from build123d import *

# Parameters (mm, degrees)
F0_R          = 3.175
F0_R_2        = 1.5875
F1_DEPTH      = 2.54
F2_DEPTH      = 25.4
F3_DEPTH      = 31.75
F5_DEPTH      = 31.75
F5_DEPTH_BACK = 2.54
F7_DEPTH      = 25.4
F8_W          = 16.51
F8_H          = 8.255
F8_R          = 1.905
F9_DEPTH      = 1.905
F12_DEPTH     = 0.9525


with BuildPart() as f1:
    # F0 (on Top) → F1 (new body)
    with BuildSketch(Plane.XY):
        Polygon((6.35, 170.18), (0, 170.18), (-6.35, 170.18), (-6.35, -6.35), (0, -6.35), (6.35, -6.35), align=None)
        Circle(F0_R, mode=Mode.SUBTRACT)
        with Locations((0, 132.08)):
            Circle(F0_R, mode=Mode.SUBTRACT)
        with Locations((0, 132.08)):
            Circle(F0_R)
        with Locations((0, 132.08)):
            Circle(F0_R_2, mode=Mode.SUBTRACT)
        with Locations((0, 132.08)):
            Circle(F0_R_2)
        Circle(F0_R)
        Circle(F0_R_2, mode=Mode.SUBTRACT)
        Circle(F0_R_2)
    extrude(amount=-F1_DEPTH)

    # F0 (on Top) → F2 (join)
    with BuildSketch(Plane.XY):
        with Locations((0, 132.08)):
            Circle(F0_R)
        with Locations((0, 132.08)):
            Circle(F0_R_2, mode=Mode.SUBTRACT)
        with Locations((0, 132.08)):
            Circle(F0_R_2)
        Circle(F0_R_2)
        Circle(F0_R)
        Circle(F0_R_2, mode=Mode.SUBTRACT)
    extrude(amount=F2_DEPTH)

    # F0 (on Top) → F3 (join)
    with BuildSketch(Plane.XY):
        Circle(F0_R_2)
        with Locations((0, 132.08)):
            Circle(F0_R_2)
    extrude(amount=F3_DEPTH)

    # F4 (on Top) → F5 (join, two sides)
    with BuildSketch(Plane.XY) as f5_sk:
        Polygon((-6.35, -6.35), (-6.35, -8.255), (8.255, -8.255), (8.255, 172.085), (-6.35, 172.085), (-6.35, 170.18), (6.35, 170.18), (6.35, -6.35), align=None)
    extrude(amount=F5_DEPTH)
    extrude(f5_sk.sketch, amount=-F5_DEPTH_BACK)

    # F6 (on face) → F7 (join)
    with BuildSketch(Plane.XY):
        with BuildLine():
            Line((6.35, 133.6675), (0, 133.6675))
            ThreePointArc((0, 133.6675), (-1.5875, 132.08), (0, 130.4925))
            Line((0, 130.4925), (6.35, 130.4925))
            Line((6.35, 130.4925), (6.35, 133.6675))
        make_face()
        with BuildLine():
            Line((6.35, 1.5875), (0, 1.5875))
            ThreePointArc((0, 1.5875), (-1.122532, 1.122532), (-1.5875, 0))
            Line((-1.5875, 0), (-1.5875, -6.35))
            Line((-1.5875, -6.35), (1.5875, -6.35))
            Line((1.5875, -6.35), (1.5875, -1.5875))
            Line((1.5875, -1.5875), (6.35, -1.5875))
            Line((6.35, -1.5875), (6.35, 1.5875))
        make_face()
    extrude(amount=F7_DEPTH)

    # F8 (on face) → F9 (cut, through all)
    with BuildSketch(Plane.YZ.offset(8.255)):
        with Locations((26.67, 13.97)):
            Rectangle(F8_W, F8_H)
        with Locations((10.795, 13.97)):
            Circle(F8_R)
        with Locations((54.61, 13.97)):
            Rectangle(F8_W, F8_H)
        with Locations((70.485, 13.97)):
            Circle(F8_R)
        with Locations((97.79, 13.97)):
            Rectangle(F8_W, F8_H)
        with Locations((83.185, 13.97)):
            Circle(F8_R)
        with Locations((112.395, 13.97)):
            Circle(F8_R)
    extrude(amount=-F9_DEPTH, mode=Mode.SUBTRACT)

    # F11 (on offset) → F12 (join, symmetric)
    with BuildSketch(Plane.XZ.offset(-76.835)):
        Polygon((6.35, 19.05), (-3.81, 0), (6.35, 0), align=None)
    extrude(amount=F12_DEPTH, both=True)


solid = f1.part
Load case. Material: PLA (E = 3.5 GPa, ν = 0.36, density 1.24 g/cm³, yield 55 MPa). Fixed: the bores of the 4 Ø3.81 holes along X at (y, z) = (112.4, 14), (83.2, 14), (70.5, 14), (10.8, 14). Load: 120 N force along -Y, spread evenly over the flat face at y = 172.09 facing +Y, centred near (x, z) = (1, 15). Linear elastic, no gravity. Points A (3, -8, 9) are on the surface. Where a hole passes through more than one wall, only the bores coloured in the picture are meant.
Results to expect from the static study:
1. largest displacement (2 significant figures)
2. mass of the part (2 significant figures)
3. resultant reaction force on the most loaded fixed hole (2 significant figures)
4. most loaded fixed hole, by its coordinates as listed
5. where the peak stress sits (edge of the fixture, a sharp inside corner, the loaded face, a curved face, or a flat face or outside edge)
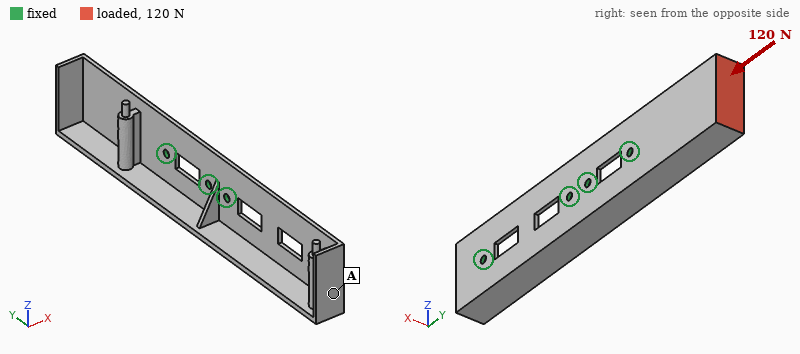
1.9 mm
26 g
55 N
(112.4, 14)
the loaded face
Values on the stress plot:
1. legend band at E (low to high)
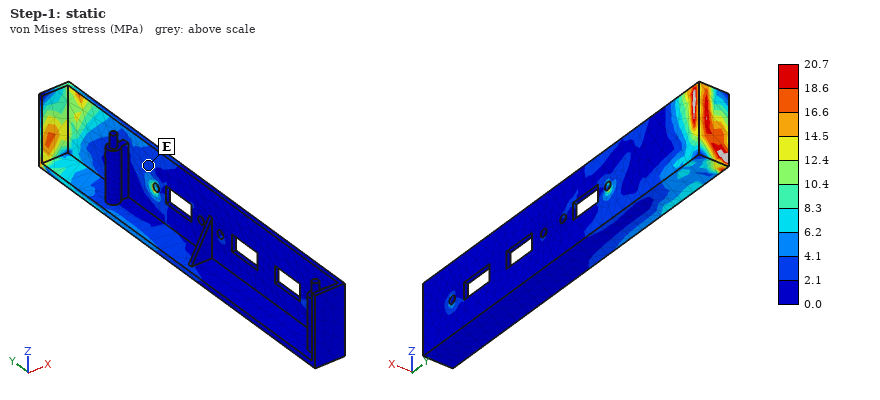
2.1 to 4.1 MPa
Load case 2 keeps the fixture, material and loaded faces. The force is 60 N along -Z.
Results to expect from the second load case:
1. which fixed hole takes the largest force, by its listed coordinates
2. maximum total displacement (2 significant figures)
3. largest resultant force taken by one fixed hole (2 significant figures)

(112.4, 14)
2.2 mm
130 N
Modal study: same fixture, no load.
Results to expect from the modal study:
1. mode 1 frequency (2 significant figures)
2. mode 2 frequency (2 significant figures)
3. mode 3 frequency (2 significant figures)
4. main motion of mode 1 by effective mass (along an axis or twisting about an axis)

320 Hz
420 Hz
670 Hz
along X
